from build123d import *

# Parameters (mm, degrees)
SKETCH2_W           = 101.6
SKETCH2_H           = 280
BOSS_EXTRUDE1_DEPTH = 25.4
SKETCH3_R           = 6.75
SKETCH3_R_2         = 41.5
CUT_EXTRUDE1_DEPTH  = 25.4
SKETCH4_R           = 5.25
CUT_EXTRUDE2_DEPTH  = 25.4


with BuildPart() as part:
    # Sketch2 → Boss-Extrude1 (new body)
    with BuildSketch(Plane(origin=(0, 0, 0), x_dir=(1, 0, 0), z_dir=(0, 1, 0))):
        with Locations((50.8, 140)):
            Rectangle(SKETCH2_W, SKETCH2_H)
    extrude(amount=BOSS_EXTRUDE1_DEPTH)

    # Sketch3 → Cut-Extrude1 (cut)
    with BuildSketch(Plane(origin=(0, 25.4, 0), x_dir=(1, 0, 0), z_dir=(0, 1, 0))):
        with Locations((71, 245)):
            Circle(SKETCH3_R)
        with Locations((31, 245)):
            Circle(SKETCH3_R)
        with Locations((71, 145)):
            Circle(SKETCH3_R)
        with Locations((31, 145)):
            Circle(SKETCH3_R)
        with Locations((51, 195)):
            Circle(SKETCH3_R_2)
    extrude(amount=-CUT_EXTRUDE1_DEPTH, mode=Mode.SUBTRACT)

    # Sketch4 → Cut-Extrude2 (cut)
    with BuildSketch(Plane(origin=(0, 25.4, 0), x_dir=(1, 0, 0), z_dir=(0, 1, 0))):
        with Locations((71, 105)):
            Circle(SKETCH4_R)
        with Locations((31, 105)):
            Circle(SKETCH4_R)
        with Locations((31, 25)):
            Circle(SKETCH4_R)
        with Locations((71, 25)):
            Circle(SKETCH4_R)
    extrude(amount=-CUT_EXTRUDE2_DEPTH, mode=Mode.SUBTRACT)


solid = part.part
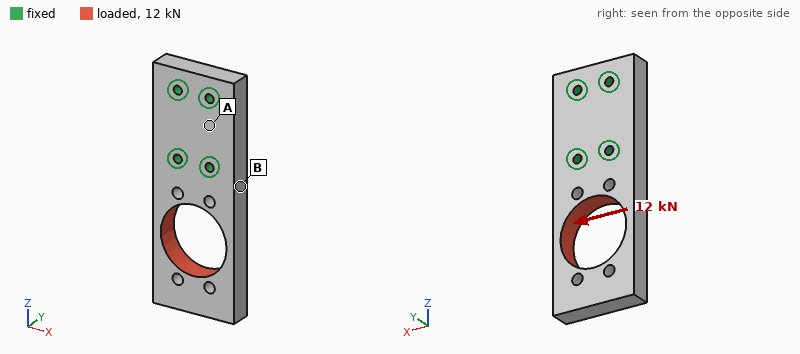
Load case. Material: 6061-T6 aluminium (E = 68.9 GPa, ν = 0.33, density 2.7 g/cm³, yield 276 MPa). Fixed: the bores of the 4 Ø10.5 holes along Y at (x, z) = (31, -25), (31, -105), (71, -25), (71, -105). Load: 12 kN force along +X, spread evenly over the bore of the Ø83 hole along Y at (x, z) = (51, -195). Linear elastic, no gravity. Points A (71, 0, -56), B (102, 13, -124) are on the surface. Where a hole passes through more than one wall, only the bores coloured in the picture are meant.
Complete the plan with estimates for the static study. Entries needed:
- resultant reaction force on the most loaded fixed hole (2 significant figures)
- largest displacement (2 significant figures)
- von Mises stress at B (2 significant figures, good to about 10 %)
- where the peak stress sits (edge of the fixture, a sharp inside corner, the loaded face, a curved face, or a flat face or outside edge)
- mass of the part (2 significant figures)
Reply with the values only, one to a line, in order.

16 kN
0.36 mm
26 MPa
a flat face or outside edge
1.5 kg
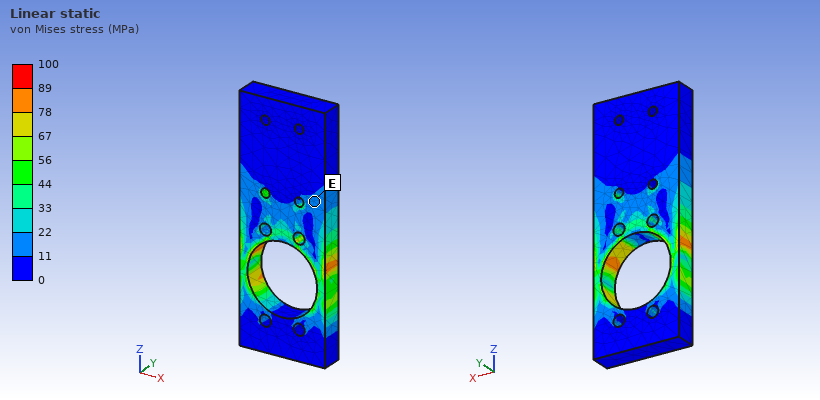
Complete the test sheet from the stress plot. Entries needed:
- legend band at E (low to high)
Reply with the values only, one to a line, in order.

11 to 22 MPa
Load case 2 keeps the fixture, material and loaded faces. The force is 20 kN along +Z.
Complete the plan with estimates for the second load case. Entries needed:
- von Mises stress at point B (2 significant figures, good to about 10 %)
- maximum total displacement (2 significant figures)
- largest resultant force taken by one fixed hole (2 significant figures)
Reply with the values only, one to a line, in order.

13 MPa
45 µm
8.4 kN
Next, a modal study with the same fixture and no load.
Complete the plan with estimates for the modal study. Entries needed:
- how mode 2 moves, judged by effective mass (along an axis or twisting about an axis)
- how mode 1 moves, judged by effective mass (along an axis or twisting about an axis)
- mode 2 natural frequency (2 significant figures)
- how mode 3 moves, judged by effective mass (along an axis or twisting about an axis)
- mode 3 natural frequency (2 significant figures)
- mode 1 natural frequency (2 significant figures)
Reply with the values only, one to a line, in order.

along X
along Y
1100 Hz
twisting about Z
1500 Hz
520 Hz
